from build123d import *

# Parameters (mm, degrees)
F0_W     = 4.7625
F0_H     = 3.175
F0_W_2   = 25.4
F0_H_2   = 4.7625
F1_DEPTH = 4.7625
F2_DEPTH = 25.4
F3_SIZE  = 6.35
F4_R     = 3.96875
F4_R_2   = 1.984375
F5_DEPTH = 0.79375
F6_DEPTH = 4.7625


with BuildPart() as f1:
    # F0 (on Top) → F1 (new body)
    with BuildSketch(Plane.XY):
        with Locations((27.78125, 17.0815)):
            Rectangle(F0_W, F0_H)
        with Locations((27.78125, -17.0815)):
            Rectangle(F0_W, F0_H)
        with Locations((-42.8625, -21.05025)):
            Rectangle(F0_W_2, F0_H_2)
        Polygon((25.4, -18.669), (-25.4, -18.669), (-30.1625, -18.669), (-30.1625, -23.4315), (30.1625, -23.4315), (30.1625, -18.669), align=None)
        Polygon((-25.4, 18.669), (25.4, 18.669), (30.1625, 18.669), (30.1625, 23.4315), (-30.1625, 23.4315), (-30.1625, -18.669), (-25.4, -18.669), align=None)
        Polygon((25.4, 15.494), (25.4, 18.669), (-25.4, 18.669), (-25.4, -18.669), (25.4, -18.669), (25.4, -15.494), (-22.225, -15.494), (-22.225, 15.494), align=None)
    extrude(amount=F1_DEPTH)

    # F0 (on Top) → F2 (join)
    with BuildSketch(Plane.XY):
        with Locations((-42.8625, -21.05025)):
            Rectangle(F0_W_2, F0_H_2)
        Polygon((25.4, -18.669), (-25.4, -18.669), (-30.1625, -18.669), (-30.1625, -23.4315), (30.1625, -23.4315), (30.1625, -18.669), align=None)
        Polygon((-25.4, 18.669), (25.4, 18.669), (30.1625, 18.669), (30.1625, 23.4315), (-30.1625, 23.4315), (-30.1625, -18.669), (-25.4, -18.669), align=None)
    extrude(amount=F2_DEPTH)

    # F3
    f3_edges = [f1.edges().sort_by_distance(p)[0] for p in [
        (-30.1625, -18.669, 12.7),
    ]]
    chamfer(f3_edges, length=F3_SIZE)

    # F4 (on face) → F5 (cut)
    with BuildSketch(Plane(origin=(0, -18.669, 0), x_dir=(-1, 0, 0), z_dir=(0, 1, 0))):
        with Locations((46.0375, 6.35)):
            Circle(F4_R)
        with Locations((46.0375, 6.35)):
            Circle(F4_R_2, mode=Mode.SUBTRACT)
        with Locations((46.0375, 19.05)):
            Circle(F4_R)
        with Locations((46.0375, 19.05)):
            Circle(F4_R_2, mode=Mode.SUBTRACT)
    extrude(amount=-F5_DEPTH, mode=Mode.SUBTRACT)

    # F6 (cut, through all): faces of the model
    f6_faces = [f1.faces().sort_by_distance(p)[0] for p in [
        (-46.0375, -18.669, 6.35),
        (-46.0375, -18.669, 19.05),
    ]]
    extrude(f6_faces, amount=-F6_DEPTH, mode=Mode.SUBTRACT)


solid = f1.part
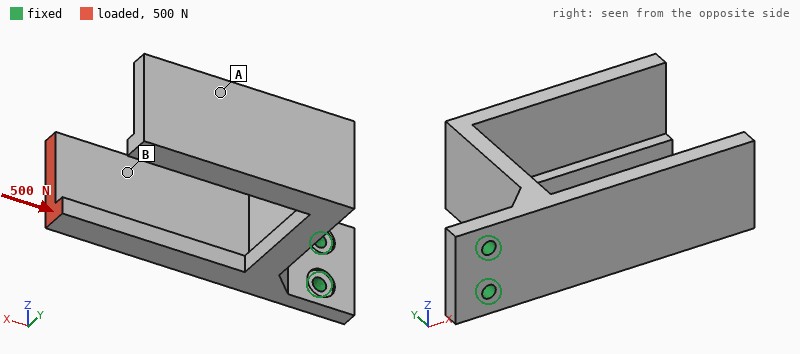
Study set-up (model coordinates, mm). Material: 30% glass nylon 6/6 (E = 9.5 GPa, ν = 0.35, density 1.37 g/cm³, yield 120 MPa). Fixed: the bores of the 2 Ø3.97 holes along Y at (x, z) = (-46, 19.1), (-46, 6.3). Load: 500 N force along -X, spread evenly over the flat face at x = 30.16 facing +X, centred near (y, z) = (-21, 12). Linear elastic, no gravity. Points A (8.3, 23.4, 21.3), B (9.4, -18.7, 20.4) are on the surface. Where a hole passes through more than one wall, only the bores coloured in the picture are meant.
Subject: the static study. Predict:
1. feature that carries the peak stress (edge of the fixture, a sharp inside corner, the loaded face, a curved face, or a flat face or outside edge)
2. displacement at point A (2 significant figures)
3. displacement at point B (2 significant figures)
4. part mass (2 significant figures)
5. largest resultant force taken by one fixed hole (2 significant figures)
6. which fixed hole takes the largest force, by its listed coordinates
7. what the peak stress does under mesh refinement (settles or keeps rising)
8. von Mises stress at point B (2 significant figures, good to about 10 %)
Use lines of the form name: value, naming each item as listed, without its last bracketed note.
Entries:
feature that carries the peak stress: edge of the fixture
displacement at point A: 0.084 mm
displacement at point B: 0.062 mm
part mass: 34 g
largest resultant force taken by one fixed hole: 290 N
which fixed hole takes the largest force, by its listed coordinates: (-46, 6.3)
what the peak stress does under mesh refinement: keeps rising
von Mises stress at point B: 3.7 MPa
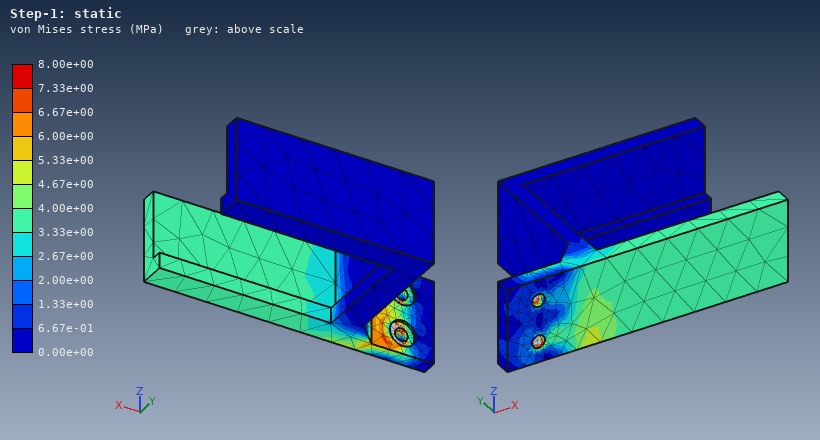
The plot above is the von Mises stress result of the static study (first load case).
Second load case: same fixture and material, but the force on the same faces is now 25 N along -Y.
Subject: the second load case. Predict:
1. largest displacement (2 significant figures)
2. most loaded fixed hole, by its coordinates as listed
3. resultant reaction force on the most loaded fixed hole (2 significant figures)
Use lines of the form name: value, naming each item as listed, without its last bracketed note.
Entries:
largest displacement: 1.1 mm
most loaded fixed hole, by its coordinates as listed: (-46, 6.3)
resultant reaction force on the most loaded fixed hole: 14 N
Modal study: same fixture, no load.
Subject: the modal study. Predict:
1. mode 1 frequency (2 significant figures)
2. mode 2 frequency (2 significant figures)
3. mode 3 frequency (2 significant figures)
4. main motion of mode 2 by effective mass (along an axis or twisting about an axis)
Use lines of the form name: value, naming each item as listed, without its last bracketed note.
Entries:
mode 1 frequency: 220 Hz
mode 2 frequency: 450 Hz
mode 3 frequency: 560 Hz
main motion of mode 2 by effective mass: along Z
